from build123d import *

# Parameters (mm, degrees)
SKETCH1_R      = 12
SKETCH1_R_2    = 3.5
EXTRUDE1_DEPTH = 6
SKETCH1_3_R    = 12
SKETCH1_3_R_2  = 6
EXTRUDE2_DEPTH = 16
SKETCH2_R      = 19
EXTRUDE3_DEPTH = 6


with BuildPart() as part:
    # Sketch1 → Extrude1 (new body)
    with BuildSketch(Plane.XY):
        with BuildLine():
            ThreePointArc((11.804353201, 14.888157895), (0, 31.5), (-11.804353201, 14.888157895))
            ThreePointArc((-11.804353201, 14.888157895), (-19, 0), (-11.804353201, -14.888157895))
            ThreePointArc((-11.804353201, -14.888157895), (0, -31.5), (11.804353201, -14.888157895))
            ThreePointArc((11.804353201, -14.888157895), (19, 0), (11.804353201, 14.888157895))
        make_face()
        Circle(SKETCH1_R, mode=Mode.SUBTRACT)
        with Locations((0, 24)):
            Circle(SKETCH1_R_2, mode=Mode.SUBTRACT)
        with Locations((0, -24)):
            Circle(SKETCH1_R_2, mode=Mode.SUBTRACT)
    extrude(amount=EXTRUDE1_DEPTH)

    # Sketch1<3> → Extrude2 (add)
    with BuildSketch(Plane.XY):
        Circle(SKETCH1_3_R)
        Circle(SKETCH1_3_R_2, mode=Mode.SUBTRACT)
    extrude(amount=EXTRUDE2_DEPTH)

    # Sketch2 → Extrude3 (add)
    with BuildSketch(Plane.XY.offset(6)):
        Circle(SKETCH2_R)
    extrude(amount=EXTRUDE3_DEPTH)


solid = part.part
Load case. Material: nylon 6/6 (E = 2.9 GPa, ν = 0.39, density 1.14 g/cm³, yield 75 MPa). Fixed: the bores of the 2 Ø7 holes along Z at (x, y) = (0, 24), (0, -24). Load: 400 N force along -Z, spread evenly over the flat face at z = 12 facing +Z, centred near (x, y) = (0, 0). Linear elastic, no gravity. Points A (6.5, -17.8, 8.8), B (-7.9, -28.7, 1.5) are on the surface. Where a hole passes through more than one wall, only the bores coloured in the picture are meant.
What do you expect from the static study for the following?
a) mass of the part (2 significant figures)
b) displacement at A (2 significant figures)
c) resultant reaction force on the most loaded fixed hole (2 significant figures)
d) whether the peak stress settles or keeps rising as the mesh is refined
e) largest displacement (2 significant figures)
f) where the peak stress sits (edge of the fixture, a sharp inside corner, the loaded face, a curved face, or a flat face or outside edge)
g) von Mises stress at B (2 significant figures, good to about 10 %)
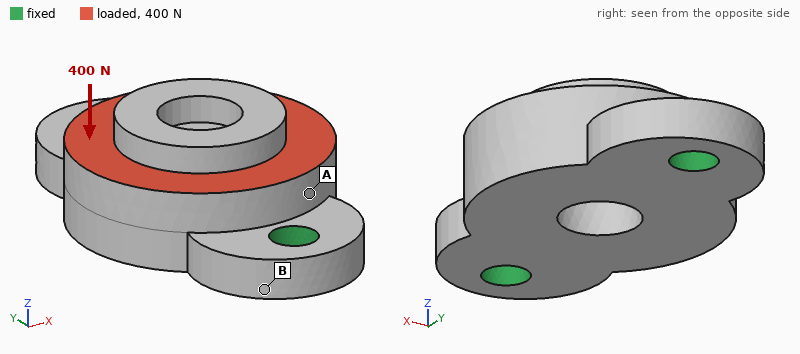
20 g
18 µm
240 N
keeps rising
46 µm
edge of the fixture
0.82 MPa
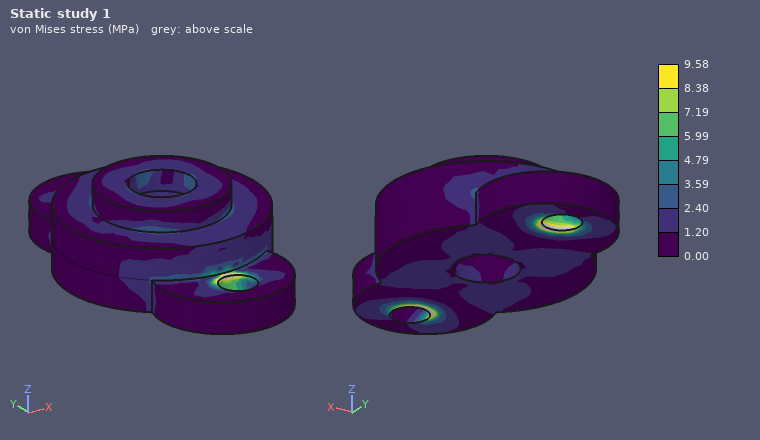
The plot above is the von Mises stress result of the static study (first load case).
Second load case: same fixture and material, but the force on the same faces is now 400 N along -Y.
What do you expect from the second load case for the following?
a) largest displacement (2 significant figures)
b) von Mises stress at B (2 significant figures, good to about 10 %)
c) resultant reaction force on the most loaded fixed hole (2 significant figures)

14 µm
0.54 MPa
220 N
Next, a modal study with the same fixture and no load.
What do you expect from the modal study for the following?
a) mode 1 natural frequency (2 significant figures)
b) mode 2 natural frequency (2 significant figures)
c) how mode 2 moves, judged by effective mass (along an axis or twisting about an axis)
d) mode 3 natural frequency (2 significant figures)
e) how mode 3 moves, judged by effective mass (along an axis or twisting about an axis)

2600 Hz
4300 Hz
along Z
6400 Hz
along X
